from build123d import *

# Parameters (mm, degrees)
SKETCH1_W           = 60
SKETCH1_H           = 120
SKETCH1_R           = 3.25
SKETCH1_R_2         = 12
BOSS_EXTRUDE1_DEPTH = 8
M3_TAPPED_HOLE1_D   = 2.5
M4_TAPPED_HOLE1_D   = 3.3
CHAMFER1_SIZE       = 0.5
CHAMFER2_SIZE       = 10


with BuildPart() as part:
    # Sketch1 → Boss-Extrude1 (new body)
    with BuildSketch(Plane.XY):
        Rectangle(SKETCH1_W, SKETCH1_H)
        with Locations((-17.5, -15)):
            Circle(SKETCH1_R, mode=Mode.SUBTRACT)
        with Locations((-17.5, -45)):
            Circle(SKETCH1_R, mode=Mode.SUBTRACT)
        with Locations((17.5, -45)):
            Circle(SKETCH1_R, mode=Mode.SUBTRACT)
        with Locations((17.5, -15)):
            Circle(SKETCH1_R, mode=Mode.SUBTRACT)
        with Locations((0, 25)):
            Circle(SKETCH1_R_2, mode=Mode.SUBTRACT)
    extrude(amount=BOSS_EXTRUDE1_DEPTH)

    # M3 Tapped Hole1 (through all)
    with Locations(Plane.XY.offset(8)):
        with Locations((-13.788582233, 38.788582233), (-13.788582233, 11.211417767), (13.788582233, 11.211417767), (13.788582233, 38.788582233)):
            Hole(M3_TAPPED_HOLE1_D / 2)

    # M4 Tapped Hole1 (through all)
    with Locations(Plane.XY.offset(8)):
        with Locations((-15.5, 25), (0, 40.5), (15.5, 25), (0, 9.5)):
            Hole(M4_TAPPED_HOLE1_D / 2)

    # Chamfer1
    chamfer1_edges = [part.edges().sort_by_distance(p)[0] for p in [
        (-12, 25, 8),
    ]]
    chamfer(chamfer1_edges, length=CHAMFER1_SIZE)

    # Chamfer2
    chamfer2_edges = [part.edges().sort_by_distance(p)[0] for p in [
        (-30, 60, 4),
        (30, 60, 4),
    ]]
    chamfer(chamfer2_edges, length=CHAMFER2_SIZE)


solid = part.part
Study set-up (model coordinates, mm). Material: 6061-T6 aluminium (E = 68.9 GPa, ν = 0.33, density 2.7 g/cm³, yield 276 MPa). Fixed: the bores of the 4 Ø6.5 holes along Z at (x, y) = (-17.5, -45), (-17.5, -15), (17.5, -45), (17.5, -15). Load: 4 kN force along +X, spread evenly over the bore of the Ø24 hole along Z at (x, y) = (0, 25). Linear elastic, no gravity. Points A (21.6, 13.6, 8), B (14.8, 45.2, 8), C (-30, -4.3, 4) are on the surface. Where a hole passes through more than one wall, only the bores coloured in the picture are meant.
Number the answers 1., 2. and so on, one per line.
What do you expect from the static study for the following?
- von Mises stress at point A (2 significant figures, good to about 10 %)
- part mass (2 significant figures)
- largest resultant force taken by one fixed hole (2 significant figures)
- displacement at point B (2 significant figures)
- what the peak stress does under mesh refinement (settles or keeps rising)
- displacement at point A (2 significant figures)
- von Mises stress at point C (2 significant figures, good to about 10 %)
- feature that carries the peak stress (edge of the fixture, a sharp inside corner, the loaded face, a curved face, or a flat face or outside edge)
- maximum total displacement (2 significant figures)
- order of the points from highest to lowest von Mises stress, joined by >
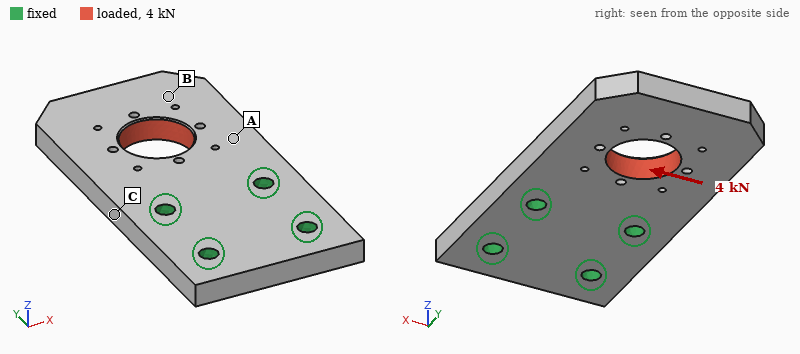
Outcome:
1. 14 MPa
2. 140 g
3. 3.9 kN
4. 49 µm
5. keeps rising
6. 22 µm
7. 25 MPa
8. edge of the fixture
9. 57 µm
10. C > A > B
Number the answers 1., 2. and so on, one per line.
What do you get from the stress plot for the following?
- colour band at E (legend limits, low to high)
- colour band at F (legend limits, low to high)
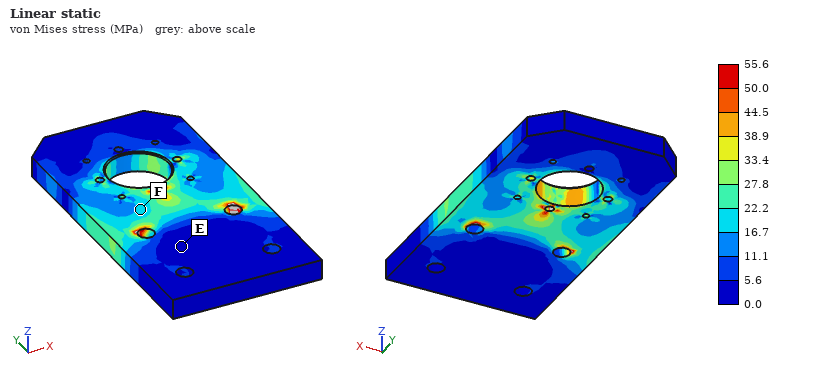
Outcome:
1. 0.0 to 5.6 MPa
2. 16.7 to 22.2 MPa
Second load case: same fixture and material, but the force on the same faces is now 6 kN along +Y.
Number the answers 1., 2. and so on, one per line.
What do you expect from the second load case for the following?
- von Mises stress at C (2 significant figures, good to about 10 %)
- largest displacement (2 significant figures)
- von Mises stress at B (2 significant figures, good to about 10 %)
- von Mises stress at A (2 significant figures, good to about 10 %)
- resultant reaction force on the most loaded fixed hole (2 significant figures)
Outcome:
1. 11 MPa
2. 26 µm
3. 8.4 MPa
4. 11 MPa
5. 2.6 kN
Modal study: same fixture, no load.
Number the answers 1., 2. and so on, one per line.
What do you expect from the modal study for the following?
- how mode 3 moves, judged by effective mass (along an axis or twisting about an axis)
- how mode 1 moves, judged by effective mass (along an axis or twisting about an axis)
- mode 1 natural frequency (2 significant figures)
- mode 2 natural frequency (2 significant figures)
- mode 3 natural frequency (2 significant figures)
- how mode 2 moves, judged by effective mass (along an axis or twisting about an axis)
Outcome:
1. along X
2. along Z
3. 1200 Hz
4. 3100 Hz
5. 5400 Hz
6. twisting about Y
